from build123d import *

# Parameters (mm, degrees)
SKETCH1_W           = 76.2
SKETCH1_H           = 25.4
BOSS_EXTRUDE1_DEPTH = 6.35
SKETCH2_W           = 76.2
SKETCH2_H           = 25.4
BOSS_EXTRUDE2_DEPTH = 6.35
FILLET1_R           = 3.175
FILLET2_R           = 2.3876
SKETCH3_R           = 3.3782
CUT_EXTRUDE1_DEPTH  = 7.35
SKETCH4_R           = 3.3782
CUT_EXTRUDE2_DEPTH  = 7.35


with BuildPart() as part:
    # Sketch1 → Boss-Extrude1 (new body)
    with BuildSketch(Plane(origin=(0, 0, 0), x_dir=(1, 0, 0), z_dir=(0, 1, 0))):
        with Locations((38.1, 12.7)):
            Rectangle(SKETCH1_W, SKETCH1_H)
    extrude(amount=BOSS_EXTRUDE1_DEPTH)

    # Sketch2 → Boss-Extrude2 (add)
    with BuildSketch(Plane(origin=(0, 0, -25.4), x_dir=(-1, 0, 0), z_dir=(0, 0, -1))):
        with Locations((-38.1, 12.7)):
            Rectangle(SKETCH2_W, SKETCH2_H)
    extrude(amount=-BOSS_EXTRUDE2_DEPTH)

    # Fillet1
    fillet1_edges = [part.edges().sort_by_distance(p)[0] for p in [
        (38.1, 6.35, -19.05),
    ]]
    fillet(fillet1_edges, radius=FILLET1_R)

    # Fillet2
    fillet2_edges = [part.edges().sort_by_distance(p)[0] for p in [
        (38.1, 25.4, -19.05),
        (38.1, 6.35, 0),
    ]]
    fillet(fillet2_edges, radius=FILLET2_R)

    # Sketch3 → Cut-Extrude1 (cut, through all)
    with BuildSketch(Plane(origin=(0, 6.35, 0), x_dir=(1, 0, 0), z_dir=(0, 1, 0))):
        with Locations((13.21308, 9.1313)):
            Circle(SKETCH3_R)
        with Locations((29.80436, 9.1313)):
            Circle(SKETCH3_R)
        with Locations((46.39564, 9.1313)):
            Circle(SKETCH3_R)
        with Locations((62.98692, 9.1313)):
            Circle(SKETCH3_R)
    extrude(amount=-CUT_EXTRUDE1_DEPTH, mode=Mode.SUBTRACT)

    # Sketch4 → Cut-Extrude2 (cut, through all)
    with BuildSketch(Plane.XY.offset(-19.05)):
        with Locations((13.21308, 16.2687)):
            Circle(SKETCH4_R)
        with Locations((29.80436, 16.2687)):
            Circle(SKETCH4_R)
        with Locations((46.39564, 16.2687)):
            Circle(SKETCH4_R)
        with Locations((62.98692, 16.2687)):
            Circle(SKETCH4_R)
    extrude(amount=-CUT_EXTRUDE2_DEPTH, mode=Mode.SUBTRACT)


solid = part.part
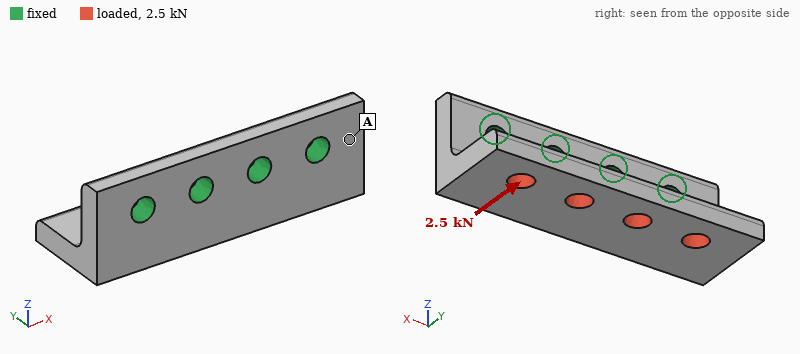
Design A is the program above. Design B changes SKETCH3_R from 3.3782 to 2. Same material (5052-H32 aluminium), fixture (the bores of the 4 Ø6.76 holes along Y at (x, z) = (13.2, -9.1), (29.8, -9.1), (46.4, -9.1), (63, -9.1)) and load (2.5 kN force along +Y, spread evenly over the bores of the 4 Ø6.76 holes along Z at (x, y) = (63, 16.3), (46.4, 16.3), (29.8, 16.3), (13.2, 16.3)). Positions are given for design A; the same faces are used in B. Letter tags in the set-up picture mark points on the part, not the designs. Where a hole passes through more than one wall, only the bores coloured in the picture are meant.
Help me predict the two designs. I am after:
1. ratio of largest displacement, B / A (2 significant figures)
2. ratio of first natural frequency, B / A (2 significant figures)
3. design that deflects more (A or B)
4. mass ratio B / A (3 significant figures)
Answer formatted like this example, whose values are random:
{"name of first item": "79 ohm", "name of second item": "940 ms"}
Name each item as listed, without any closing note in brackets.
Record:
{"ratio of largest displacement, B / A": "1.4", "ratio of first natural frequency, B / A": "0.88", "design that deflects more": "B", "mass ratio B / A": "1.03"}
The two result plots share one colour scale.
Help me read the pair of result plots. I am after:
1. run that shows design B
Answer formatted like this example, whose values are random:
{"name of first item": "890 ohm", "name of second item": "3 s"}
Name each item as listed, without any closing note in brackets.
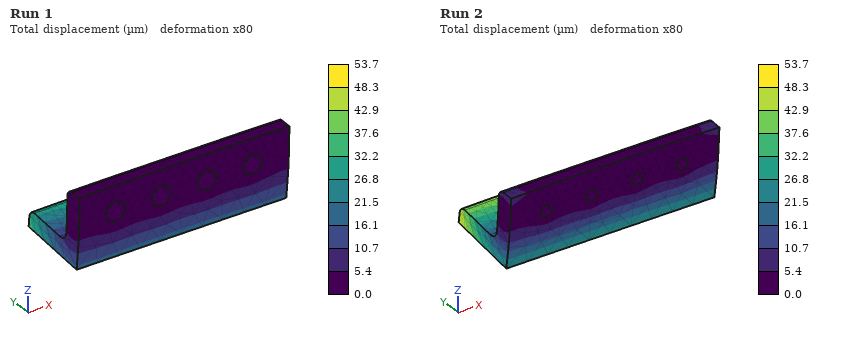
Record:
{"run that shows design B": "Run 2"}
